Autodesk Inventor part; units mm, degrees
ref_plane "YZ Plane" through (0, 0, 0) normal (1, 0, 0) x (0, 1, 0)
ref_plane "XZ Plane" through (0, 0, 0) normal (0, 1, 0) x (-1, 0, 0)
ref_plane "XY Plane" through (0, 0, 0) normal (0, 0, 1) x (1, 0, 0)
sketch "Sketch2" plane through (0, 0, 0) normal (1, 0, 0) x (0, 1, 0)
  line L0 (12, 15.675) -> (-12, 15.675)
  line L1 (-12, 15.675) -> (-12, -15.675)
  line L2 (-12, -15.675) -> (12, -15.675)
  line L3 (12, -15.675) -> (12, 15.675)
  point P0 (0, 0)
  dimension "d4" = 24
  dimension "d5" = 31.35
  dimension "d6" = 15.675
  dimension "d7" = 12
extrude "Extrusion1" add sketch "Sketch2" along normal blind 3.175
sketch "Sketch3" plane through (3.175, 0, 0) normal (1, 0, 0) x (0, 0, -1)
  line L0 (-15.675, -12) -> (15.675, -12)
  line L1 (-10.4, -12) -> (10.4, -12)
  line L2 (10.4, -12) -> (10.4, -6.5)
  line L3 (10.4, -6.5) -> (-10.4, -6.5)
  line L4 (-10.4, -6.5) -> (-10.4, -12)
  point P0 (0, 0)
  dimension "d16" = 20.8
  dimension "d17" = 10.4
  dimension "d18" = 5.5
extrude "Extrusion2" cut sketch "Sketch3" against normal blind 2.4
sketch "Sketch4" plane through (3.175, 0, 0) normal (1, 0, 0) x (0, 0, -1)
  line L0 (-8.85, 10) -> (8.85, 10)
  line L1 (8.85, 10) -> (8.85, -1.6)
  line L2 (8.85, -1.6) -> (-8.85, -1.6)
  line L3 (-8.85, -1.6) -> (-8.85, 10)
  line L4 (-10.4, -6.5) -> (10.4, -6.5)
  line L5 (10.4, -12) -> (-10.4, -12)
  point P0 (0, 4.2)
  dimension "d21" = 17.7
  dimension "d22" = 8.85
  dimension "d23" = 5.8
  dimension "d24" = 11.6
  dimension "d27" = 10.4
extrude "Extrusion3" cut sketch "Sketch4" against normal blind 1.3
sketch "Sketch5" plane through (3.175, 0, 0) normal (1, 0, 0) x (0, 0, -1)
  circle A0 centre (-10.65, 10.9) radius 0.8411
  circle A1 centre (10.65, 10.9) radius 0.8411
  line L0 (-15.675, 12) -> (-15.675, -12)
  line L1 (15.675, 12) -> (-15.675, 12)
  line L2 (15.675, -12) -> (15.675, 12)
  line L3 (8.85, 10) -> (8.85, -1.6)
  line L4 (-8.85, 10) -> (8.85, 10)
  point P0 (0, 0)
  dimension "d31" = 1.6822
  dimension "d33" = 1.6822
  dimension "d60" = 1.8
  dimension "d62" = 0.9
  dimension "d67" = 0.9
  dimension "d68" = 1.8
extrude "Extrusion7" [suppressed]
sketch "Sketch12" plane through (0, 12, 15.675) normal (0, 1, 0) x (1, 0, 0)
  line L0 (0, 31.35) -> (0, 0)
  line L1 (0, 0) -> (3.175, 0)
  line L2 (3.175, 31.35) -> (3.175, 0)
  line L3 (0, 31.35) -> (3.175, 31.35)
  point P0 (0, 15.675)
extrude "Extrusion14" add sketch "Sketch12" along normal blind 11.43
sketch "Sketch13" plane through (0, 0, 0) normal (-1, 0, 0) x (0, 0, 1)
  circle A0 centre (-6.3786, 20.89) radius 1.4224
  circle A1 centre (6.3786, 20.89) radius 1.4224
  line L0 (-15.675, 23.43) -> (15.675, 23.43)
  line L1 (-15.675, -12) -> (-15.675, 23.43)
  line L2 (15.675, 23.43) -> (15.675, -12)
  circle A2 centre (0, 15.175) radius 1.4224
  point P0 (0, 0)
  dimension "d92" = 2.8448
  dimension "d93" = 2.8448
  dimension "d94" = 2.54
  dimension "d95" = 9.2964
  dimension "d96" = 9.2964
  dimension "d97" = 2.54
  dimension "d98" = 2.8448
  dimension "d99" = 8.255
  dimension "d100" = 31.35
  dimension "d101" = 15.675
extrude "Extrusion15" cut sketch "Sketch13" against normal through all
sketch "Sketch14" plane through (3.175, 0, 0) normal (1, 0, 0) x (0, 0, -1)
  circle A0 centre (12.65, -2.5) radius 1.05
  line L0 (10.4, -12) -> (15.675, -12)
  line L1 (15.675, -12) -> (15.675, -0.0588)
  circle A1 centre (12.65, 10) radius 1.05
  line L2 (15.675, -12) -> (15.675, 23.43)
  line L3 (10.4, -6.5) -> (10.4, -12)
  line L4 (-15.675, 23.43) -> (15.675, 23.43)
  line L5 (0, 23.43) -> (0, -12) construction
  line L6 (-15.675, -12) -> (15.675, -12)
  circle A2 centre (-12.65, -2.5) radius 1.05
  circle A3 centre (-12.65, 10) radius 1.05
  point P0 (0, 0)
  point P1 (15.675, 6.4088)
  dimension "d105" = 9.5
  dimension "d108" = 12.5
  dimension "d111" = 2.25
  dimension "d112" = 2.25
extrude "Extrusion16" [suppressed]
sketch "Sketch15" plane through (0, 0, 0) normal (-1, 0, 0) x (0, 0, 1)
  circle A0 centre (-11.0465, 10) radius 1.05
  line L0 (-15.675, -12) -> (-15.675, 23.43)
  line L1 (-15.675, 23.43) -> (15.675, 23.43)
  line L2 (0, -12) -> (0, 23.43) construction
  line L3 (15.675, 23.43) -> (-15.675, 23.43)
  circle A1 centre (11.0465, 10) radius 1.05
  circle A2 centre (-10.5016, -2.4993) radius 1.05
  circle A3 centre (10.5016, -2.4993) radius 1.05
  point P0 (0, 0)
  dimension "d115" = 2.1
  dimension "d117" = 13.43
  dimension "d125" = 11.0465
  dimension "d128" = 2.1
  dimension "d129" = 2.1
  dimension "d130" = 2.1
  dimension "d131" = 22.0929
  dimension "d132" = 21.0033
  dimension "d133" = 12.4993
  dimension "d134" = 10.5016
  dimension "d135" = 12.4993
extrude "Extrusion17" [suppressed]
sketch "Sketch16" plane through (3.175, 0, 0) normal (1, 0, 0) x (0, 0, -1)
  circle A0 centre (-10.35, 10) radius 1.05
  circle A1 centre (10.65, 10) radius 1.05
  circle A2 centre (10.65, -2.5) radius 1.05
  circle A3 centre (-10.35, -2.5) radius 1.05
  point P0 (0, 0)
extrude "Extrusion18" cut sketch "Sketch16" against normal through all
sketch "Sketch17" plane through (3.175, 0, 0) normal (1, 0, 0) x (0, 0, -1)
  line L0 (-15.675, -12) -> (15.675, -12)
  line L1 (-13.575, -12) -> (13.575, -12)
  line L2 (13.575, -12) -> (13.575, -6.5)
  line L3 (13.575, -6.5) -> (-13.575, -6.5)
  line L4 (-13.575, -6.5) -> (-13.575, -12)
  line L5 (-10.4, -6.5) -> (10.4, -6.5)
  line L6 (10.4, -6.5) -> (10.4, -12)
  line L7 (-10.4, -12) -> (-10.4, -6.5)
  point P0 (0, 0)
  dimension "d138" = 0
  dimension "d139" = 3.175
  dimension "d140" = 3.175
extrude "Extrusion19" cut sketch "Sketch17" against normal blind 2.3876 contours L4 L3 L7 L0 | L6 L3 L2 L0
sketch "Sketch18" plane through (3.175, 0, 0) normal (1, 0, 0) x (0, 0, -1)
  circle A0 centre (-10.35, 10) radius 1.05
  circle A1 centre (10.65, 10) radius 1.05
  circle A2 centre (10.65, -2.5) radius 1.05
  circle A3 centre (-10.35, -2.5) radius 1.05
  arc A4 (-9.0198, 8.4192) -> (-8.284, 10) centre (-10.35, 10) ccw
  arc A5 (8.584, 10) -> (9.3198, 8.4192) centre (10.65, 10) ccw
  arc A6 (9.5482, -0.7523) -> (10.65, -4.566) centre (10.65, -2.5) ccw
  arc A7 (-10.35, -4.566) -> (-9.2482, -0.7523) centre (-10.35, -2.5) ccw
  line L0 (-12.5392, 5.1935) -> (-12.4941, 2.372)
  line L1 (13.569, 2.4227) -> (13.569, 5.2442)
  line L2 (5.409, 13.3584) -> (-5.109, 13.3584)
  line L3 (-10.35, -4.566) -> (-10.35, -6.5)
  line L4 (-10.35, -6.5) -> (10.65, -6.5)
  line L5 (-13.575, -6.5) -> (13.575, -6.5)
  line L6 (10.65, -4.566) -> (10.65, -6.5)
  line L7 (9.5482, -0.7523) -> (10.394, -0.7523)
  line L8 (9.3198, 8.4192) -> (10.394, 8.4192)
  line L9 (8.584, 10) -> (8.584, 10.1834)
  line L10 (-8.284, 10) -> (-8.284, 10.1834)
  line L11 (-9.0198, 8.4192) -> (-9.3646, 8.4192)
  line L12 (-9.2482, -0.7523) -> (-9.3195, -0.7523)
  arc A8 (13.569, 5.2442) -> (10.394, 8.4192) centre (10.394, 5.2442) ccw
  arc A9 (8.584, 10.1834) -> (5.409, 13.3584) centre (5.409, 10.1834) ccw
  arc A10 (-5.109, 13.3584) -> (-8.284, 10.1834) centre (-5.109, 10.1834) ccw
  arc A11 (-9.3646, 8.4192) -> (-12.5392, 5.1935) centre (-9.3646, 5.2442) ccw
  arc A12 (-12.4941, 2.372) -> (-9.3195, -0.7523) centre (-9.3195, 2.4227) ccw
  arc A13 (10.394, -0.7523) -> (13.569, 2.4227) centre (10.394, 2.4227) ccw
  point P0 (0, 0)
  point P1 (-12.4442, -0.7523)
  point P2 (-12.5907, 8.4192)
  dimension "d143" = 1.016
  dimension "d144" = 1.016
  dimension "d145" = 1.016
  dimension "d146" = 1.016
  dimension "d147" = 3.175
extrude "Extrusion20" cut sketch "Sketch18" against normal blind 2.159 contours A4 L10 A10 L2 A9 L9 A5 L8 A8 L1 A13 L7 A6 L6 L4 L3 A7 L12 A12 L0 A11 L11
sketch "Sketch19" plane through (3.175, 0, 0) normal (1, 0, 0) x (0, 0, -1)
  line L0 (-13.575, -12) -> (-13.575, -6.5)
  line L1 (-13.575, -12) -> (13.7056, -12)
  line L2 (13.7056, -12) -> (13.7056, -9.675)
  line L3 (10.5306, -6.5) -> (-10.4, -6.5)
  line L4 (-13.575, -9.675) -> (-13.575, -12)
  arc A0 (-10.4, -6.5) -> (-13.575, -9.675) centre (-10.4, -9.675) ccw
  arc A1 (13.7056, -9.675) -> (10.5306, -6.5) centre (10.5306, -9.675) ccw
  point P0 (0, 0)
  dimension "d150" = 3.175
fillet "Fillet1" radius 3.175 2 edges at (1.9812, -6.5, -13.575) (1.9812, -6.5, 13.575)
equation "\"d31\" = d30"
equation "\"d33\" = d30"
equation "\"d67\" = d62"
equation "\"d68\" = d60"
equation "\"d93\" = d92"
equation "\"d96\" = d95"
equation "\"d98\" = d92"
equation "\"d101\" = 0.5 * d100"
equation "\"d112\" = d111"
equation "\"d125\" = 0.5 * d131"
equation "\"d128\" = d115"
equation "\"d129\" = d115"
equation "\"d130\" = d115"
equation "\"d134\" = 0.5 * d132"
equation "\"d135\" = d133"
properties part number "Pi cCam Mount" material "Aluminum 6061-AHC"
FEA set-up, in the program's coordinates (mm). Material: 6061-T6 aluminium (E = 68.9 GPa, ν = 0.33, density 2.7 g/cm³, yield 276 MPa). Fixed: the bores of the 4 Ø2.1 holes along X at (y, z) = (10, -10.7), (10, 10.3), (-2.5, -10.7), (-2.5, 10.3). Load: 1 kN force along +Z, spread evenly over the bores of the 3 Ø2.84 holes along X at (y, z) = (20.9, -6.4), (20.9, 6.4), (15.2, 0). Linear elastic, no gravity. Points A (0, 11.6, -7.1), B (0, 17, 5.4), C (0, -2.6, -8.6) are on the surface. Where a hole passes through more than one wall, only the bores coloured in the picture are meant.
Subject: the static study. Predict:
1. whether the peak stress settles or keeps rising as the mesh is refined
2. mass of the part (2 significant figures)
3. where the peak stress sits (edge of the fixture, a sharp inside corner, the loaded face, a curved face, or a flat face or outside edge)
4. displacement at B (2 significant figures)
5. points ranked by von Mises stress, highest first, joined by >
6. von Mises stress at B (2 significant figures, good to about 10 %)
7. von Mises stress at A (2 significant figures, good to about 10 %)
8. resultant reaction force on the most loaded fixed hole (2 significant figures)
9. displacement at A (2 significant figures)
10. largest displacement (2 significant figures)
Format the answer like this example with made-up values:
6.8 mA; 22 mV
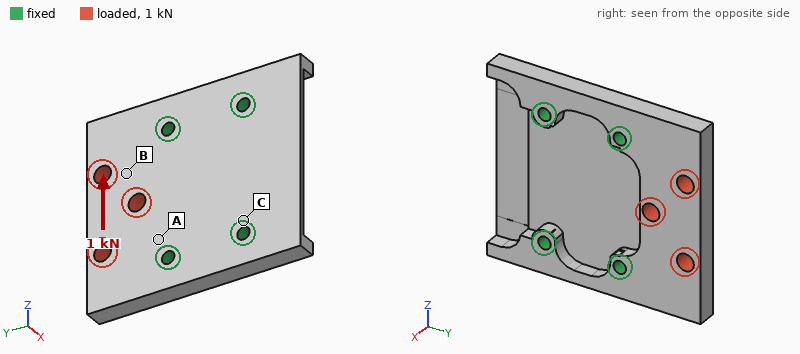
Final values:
keeps rising; 5.9 g; edge of the fixture; 6.1 µm; A > B > C; 21 MPa; 41 MPa; 580 N; 2.2 µm; 10 µm
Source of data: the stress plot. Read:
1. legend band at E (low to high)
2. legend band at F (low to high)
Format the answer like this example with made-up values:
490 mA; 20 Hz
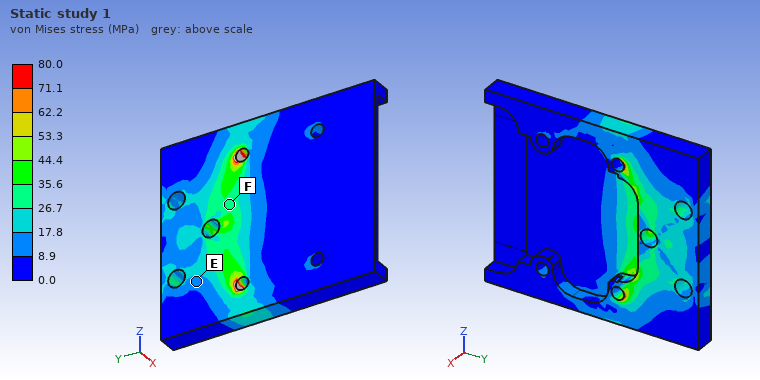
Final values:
8.9 to 17.8 MPa; 26.7 to 35.6 MPa
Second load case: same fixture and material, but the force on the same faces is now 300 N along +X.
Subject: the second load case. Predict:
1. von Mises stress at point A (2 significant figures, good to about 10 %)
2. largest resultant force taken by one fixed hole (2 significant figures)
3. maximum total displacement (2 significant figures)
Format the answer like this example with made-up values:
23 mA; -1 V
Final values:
48 MPa; 180 N; 54 µm
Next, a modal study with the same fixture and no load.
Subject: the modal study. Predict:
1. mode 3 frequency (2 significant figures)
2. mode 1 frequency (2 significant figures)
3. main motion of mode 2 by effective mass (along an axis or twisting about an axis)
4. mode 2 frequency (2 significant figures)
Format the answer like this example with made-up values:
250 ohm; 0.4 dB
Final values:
17 kHz; 10 kHz; along X; 11 kHz
